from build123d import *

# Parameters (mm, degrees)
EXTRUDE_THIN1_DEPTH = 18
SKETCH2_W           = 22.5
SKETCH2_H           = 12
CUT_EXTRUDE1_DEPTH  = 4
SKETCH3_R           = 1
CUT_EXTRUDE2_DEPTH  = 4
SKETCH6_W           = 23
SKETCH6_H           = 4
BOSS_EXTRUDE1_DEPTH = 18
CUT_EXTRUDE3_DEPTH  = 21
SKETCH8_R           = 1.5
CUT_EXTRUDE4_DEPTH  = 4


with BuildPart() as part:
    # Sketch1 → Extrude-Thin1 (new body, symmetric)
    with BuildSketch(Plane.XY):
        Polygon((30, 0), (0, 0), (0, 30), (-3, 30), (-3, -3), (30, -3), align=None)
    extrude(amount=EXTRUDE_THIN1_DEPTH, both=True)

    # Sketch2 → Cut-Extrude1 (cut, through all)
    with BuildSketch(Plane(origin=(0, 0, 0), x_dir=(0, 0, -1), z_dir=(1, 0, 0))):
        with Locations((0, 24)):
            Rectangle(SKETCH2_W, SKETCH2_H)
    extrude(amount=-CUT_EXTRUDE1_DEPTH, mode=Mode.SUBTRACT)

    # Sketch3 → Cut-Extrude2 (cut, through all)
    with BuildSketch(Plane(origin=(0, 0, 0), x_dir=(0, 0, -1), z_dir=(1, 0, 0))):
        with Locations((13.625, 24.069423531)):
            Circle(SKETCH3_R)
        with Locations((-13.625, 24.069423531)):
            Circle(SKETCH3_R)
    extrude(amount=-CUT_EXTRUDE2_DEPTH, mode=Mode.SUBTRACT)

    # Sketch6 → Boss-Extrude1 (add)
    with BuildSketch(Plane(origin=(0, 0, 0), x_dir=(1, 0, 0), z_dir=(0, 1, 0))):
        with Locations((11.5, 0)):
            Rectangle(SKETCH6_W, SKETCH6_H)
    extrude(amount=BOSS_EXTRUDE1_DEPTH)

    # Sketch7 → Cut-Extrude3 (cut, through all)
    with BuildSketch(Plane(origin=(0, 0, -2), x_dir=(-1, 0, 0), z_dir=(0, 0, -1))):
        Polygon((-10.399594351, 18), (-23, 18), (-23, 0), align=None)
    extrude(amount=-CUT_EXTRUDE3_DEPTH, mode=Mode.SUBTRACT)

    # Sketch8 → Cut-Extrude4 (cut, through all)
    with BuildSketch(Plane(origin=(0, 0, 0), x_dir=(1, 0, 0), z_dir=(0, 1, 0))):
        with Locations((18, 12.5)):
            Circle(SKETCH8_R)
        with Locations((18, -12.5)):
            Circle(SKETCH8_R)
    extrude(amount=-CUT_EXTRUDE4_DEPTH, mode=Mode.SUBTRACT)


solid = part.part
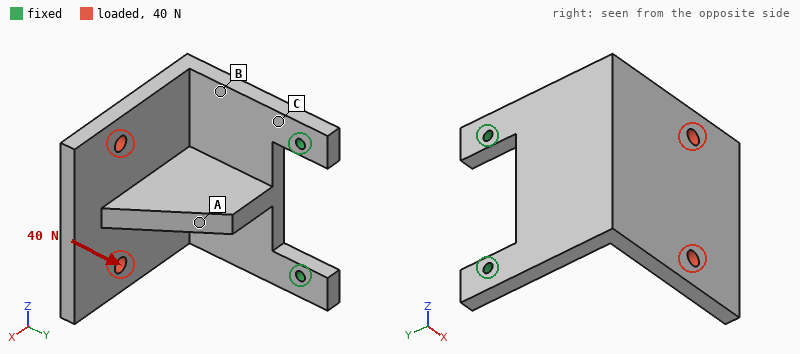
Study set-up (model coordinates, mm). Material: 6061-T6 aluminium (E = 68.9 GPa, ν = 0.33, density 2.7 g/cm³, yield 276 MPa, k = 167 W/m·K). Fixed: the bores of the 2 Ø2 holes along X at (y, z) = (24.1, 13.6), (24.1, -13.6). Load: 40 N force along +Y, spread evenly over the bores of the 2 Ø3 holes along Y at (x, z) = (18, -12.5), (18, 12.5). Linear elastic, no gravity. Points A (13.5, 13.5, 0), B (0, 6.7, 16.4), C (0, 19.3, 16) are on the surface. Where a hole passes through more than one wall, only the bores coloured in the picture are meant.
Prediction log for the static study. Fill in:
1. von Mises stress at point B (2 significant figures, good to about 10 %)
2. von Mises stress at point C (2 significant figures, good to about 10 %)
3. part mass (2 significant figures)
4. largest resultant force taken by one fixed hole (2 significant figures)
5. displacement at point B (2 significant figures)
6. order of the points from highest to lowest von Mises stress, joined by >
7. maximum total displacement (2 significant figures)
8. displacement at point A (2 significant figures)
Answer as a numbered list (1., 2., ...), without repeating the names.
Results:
1. 9.0 MPa
2. 36 MPa
3. 19 g
4. 20 N
5. 0.047 mm
6. C > B > A
7. 0.17 mm
8. 0.070 mm
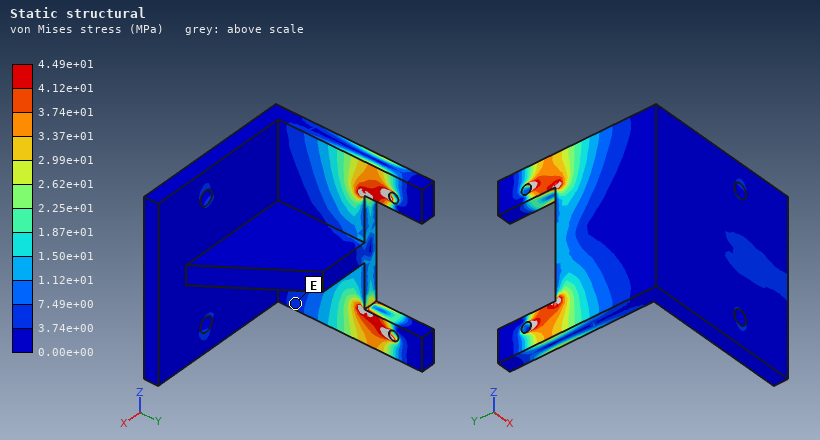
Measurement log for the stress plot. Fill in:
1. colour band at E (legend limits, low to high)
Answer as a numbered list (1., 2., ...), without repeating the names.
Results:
1. 3.74e+00 to 7.49e+00 MPa
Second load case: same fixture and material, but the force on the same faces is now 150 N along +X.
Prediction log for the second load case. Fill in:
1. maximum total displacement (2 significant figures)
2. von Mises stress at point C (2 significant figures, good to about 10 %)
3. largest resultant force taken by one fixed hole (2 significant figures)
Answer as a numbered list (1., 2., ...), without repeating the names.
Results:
1. 0.62 mm
2. 140 MPa
3. 75 N
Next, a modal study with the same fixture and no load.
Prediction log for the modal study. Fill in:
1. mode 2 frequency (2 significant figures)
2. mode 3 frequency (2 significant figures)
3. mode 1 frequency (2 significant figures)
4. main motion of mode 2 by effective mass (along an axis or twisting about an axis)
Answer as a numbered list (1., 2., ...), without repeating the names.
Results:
1. 2000 Hz
2. 4000 Hz
3. 740 Hz
4. along Z
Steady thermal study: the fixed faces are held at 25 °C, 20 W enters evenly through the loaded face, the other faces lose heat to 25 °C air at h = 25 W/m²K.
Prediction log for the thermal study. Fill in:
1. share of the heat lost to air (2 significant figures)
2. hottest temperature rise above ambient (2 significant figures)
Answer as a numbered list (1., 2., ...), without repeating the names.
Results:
1. 22 %
2. 53 K
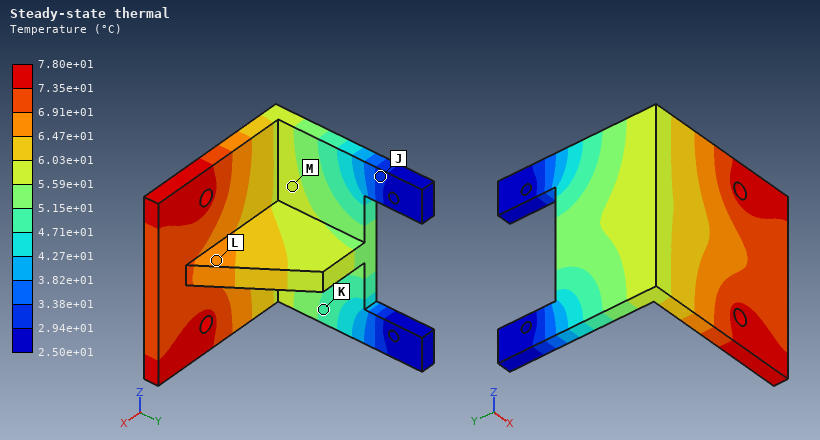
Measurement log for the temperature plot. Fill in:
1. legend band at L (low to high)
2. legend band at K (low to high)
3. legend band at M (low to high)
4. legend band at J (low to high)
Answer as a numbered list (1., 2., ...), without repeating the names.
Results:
1. 6.47e+01 to 6.91e+01 °C
2. 4.71e+01 to 5.15e+01 °C
3. 5.59e+01 to 6.03e+01 °C
4. 2.94e+01 to 3.38e+01 °C
